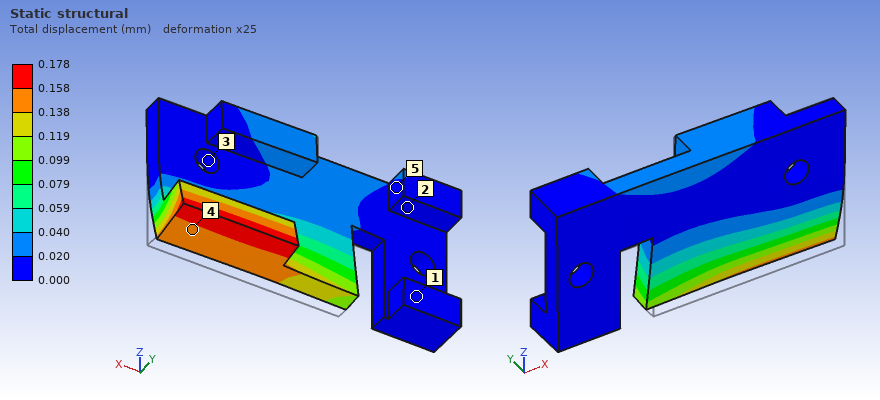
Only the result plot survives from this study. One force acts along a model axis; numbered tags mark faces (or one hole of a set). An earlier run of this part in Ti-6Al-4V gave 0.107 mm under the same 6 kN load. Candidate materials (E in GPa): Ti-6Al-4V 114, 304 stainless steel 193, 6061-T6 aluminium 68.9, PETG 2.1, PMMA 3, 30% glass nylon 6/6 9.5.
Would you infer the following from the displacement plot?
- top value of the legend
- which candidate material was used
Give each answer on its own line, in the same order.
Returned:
0.178 mm
6061-T6 aluminium
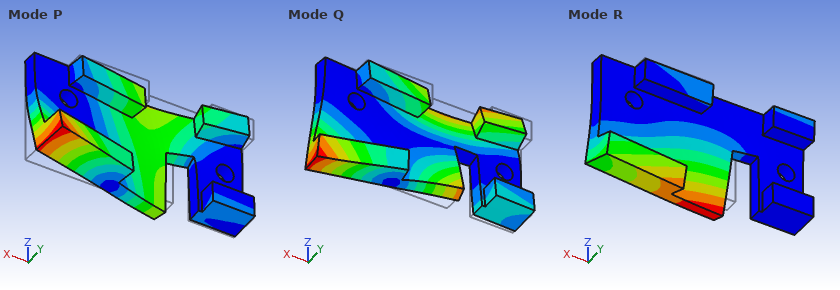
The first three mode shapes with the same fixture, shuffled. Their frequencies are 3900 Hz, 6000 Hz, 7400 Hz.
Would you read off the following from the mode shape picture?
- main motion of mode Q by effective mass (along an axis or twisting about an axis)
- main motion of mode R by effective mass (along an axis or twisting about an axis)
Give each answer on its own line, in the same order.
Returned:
along Y
along Y
